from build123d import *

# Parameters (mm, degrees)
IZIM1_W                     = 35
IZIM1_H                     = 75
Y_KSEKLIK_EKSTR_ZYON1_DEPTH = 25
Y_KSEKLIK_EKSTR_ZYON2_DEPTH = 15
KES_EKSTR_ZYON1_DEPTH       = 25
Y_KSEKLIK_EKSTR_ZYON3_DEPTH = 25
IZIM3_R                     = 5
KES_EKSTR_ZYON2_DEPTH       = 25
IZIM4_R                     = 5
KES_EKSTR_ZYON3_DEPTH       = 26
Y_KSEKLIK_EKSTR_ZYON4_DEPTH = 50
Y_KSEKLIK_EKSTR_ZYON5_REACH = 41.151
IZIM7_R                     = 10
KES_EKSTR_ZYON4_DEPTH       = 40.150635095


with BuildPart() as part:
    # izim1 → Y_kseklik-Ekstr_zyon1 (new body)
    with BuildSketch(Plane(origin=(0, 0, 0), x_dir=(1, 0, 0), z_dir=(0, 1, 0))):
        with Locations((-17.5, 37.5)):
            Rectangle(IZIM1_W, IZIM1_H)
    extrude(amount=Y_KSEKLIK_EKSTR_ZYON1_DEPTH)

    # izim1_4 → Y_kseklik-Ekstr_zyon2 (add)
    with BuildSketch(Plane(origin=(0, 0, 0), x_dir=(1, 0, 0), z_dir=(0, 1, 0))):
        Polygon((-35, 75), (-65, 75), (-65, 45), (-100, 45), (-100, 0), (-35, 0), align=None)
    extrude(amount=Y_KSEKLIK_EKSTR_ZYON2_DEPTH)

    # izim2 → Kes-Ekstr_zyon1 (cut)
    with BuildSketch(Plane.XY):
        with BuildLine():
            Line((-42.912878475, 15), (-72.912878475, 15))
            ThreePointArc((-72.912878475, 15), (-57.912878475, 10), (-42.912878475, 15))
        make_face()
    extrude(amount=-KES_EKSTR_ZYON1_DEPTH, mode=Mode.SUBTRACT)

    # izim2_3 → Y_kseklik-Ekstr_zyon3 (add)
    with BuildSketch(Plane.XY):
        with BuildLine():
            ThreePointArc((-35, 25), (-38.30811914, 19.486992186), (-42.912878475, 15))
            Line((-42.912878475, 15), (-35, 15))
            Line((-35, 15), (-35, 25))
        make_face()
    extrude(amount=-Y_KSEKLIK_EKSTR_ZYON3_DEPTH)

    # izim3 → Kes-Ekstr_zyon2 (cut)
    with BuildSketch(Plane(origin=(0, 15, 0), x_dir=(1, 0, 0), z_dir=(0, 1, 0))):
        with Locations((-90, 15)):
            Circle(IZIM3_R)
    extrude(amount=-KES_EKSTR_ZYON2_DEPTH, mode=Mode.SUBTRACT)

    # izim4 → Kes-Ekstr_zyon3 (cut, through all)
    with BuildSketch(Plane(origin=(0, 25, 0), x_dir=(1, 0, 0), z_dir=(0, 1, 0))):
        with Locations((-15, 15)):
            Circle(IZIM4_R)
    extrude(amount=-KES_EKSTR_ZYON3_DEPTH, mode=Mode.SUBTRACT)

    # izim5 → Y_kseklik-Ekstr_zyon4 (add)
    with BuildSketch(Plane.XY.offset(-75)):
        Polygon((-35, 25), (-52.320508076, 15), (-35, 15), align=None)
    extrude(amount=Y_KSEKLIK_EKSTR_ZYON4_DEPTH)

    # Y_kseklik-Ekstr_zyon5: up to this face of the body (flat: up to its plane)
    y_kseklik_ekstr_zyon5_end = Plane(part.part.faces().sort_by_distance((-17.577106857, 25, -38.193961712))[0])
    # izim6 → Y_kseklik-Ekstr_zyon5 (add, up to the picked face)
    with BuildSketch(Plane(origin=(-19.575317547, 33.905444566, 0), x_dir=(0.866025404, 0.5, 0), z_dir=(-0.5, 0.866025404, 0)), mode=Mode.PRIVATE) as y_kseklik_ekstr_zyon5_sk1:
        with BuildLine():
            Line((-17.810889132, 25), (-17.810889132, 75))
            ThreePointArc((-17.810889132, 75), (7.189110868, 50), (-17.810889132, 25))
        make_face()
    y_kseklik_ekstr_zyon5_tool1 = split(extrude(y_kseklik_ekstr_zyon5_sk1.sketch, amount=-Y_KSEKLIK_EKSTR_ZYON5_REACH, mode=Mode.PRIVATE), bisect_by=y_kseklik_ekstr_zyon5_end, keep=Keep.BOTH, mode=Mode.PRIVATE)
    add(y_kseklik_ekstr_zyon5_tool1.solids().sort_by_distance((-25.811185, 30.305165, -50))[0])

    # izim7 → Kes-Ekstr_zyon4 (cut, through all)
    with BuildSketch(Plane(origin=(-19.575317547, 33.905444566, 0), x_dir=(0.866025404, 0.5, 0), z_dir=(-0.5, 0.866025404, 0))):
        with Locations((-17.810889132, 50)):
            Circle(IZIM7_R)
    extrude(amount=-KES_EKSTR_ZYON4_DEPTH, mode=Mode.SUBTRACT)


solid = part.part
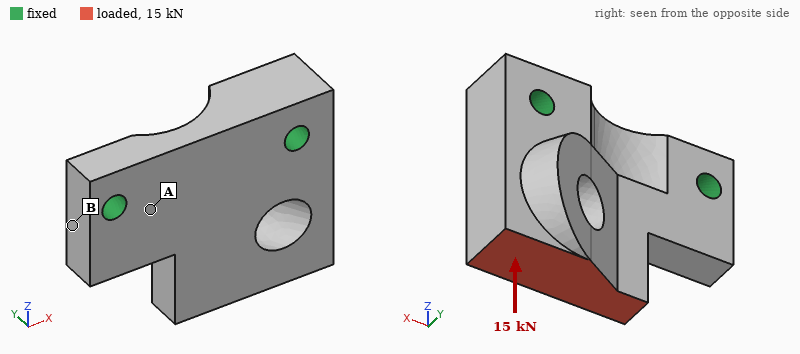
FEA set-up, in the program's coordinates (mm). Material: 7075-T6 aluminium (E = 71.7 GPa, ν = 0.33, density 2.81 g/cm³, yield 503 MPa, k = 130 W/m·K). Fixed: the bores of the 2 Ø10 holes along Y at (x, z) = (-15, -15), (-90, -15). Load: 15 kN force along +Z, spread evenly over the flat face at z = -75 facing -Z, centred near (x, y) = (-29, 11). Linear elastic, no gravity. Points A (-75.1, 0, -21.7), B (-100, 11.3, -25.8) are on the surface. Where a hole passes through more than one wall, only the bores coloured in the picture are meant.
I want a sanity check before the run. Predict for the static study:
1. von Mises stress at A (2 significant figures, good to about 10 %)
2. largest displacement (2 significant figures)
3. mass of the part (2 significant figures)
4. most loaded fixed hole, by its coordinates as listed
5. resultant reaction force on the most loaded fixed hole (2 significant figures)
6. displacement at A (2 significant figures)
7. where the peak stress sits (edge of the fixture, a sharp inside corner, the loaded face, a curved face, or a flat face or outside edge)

14 MPa
20 µm
340 g
(-15, -15)
12 kN
4.3 µm
a curved face
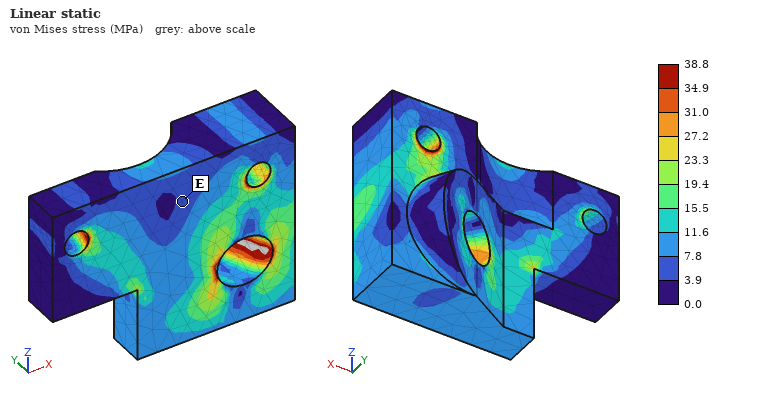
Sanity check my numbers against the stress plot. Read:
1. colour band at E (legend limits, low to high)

3.9 to 7.8 MPa
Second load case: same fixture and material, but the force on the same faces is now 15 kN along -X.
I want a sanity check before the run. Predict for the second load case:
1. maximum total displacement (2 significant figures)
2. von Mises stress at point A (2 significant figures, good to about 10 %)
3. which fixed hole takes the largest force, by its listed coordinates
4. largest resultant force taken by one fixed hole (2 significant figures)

93 µm
41 MPa
(-90, -15)
14 kN
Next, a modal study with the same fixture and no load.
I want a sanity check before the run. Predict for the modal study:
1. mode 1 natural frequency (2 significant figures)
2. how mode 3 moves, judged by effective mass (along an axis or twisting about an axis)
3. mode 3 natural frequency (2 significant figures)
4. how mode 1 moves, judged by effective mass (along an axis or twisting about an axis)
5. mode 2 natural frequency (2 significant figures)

4100 Hz
along X
8500 Hz
along Y
7700 Hz
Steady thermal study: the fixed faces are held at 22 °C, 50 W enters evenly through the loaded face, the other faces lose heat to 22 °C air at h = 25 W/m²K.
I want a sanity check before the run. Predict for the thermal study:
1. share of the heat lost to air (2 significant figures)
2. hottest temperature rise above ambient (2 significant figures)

6.3 %
19 K
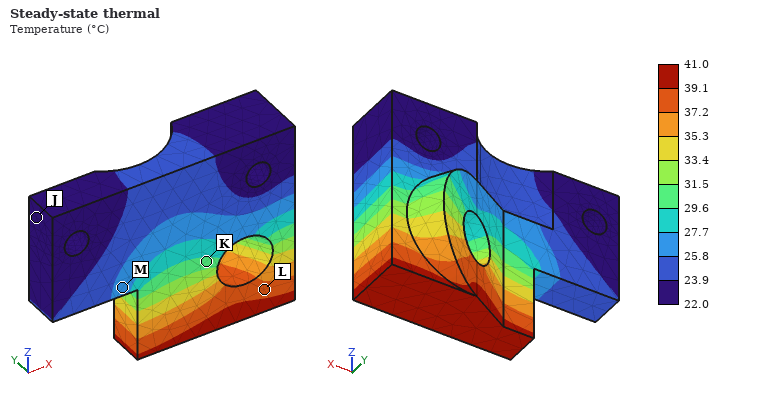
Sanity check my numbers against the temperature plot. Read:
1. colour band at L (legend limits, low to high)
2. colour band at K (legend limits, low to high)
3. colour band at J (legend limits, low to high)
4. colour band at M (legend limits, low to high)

37.2 to 39.1 °C
29.6 to 31.5 °C
22.0 to 23.9 °C
25.8 to 27.7 °C
